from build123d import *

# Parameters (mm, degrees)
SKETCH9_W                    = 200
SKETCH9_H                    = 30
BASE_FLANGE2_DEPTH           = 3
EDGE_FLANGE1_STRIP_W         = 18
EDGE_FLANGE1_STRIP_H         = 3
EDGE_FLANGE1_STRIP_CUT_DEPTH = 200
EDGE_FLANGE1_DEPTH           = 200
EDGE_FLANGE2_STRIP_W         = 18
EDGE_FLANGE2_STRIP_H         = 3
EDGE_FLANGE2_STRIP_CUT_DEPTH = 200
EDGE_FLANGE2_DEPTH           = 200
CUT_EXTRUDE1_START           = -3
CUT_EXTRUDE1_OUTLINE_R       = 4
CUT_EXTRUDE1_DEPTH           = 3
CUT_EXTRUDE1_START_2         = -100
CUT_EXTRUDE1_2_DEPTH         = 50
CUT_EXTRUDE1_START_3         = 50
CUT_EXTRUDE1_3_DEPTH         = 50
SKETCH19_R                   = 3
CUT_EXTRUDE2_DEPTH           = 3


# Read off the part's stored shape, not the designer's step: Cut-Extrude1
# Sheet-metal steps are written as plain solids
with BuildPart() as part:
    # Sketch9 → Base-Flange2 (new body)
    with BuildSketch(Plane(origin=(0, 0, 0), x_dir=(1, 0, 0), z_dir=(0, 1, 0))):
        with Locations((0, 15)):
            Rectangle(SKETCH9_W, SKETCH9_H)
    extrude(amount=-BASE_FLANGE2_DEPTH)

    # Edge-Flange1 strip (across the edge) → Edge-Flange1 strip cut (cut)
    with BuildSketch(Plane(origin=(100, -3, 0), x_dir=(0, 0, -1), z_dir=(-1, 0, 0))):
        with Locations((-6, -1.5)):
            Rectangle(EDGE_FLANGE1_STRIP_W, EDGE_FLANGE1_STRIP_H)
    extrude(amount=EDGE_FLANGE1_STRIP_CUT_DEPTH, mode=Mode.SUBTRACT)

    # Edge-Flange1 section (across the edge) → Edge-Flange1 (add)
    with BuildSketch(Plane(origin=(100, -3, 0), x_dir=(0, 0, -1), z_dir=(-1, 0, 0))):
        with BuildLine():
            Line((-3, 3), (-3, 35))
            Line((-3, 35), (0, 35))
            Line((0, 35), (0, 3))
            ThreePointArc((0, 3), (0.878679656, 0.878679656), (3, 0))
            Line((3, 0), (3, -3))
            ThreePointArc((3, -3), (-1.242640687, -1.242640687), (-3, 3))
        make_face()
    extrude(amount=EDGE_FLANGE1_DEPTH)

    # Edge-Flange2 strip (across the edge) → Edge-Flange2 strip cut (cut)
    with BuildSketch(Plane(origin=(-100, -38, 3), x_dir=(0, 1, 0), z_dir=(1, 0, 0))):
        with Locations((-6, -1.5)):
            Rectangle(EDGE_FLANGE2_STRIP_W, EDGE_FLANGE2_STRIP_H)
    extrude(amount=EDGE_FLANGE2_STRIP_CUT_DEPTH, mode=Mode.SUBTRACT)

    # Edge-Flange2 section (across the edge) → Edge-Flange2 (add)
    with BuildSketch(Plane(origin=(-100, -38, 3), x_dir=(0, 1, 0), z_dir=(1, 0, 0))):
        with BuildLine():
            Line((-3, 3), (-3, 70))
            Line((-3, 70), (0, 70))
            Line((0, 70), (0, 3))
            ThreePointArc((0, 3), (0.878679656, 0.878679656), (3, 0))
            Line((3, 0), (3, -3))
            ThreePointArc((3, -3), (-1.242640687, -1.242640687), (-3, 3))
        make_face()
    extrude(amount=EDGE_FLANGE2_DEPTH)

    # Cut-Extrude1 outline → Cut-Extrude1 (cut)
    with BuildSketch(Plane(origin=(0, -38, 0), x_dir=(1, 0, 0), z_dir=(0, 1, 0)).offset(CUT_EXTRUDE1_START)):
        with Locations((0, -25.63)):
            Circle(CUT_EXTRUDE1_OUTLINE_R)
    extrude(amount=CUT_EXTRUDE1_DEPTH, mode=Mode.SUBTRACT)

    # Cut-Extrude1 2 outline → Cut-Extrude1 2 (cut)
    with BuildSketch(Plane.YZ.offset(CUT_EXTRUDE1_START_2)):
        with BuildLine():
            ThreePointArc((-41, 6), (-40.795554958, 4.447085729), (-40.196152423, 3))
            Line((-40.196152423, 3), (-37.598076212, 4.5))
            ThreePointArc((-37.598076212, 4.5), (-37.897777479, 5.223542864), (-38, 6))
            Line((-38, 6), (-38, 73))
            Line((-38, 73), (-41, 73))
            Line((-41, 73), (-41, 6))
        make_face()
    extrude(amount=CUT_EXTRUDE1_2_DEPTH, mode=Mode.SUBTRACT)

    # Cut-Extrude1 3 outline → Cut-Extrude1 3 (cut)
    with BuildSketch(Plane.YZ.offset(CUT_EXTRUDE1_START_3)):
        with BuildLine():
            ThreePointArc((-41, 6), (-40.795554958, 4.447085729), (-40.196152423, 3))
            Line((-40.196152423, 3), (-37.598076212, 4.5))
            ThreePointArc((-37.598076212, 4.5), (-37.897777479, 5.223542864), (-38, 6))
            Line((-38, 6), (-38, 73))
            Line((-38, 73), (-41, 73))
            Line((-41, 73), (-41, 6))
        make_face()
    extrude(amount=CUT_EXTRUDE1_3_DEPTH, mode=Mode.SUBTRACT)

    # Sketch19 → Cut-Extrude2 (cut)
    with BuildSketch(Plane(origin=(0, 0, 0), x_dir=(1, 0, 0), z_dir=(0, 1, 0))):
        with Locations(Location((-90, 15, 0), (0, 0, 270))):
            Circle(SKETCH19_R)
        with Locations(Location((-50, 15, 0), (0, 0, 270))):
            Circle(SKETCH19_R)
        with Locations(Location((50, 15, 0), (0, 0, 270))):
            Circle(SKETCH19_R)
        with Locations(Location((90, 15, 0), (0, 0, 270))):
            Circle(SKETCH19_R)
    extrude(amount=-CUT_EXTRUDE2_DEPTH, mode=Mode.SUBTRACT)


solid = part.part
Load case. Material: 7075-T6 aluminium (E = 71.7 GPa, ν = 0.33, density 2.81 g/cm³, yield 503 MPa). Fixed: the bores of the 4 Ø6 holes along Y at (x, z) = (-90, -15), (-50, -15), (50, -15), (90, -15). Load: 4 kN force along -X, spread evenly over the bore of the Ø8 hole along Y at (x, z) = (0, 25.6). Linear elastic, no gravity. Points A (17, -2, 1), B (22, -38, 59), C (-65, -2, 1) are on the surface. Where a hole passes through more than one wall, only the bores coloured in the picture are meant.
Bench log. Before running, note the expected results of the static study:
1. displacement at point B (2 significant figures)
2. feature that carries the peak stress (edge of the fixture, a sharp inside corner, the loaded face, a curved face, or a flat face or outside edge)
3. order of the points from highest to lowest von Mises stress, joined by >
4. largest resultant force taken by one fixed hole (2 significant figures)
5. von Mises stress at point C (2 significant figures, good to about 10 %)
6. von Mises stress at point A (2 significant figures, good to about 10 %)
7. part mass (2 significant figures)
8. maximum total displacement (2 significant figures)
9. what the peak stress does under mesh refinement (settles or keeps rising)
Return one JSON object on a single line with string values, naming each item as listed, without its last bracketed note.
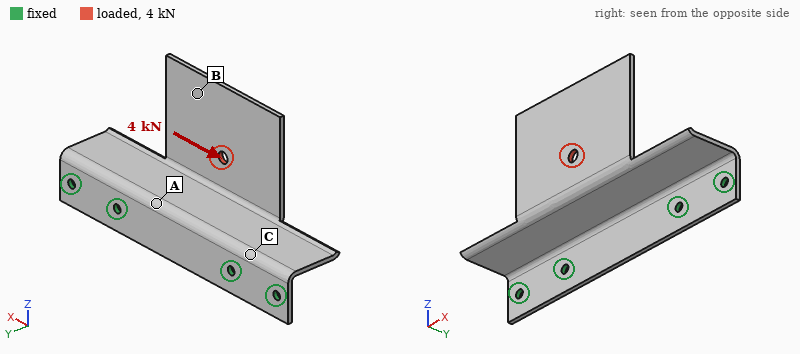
{"displacement at point B": "1.7 mm", "feature that carries the peak stress": "a sharp inside corner", "order of the points from highest to lowest von Mises stress, joined by >": "C > A > B", "largest resultant force taken by one fixed hole": "2.0 kN", "von Mises stress at point C": "140 MPa", "von Mises stress at point A": "71 MPa", "part mass": "170 g", "maximum total displacement": "2.6 mm", "what the peak stress does under mesh refinement": "keeps rising"}
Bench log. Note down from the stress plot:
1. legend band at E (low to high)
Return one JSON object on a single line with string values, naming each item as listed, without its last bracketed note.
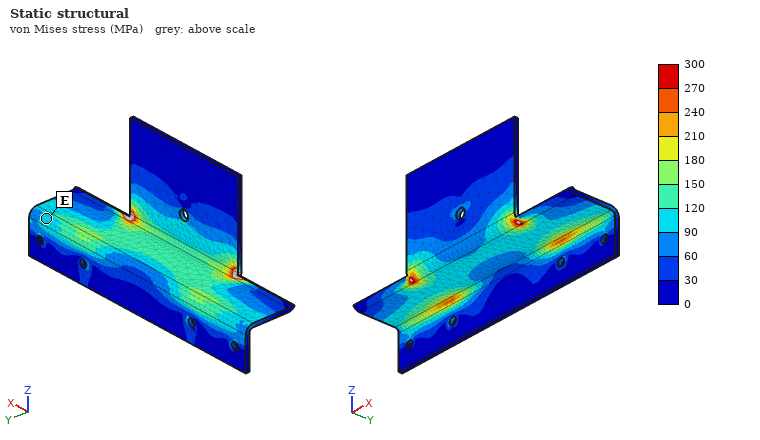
{"legend band at E": "90 to 120 MPa"}
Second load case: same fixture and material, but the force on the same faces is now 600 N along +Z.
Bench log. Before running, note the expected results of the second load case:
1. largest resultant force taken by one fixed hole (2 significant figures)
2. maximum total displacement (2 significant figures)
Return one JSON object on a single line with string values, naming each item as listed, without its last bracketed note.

{"largest resultant force taken by one fixed hole": "470 N", "maximum total displacement": "2.3 mm"}
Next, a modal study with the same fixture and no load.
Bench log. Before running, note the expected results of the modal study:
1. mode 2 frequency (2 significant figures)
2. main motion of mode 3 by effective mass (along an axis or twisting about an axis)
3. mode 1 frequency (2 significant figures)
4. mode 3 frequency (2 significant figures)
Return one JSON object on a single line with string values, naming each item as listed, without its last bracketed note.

{"mode 2 frequency": "610 Hz", "main motion of mode 3 by effective mass": "along Z", "mode 1 frequency": "250 Hz", "mode 3 frequency": "750 Hz"}
